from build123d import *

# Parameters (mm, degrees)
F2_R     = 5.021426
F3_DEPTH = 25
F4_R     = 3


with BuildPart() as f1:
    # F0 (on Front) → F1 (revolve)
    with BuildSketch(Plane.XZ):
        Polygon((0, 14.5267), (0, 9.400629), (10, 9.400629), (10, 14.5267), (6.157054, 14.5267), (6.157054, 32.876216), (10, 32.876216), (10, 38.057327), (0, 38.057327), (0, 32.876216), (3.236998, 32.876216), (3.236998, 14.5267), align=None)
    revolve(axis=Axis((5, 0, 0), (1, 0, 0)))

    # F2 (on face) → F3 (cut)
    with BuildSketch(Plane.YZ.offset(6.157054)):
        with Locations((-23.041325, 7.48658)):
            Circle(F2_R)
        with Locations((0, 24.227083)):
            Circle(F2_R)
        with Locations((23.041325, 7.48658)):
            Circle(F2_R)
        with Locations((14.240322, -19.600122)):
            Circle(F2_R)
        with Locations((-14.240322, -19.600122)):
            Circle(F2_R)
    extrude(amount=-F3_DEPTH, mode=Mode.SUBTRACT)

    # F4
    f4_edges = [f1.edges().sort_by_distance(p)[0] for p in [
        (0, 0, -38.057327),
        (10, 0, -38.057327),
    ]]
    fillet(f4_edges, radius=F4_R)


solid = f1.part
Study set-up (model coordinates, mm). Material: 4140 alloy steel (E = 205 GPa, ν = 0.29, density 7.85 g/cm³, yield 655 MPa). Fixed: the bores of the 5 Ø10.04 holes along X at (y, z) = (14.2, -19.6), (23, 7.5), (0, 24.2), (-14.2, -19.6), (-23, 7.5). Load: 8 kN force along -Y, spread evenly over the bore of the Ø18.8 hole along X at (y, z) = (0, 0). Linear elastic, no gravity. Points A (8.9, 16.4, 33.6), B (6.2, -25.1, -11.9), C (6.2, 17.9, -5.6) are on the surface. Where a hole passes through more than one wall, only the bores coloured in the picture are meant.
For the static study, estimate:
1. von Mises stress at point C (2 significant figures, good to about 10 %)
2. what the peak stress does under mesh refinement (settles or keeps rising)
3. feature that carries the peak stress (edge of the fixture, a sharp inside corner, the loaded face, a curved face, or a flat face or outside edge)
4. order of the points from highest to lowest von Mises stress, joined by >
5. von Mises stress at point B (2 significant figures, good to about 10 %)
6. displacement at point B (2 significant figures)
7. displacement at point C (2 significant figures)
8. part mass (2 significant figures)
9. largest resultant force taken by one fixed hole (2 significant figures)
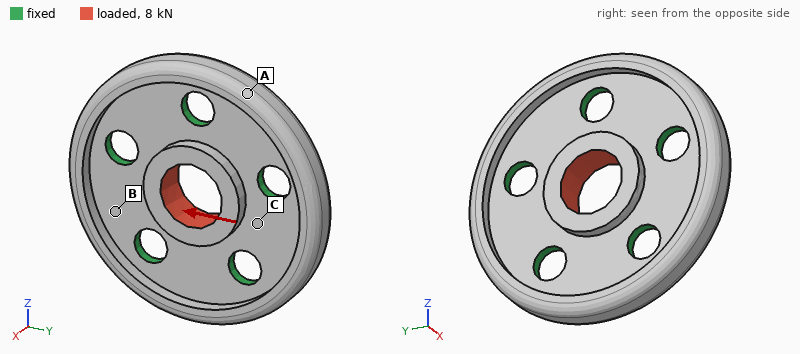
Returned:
19 MPa
keeps rising
edge of the fixture
C > B > A
9.3 MPa
0.63 µm
1.3 µm
170 g
2.2 kN
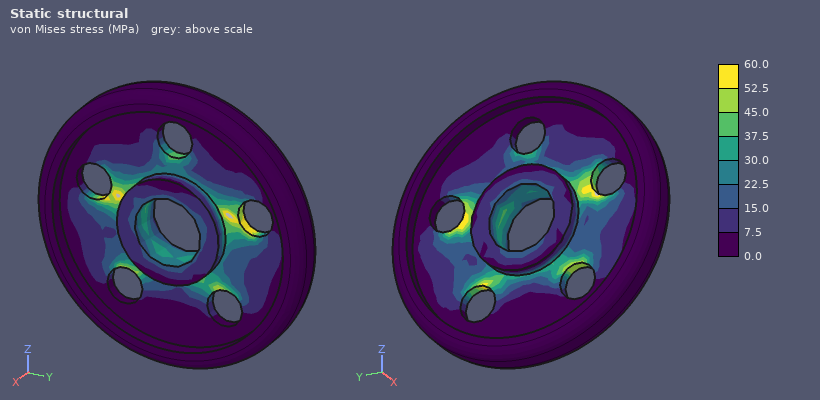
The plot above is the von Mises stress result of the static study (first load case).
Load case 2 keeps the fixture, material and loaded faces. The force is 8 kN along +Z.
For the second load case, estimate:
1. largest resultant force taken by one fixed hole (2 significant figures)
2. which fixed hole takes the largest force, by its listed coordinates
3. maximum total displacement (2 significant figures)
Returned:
2.3 kN
(0, 24.2)
2.8 µm
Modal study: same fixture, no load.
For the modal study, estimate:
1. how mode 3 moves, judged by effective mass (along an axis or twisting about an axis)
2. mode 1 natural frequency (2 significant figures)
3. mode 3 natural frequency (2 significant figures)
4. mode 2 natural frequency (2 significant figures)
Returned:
twisting about Z
11 kHz
12 kHz
11 kHz
